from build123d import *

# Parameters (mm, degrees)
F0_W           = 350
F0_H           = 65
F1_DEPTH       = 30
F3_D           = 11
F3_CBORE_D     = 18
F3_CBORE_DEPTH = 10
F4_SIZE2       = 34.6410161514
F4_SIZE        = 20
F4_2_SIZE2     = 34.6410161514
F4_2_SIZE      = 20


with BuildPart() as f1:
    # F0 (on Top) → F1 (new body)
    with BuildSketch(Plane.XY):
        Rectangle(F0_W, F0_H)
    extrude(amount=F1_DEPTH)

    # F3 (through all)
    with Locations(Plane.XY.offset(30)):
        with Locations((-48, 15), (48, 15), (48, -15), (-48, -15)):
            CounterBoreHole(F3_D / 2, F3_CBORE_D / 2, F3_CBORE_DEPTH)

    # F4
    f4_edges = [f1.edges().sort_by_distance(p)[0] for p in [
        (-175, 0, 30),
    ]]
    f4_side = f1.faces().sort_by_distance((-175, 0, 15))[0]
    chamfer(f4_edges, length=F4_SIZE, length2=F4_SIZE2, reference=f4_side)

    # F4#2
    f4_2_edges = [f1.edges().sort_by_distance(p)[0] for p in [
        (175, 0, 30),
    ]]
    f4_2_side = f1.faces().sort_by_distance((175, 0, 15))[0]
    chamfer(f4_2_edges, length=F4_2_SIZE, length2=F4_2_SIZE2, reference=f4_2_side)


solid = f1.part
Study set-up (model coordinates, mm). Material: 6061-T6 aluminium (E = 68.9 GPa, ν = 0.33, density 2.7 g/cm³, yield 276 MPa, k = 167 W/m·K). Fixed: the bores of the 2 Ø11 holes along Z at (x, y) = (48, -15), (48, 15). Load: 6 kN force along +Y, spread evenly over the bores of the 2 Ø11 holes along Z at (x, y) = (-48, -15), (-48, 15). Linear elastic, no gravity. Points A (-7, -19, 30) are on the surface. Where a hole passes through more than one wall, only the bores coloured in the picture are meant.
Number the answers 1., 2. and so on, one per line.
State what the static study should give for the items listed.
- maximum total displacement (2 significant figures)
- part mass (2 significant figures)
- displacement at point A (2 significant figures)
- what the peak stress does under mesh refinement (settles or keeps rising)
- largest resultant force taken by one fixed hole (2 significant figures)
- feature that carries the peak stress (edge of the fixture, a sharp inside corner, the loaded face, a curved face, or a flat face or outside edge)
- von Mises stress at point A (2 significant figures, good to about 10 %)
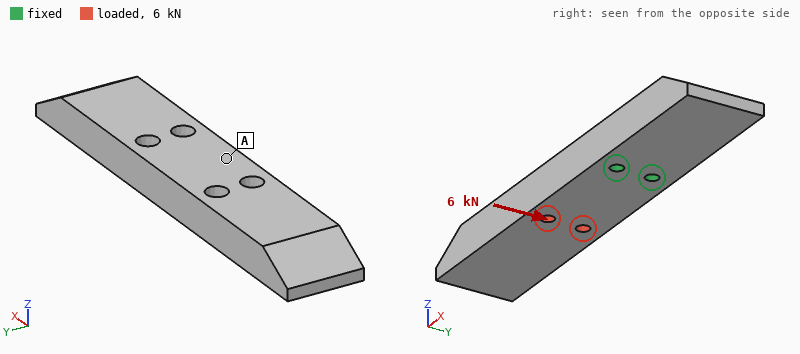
1. 0.17 mm
2. 1.7 kg
3. 0.031 mm
4. keeps rising
5. 16 kN
6. edge of the fixture
7. 6.5 MPa
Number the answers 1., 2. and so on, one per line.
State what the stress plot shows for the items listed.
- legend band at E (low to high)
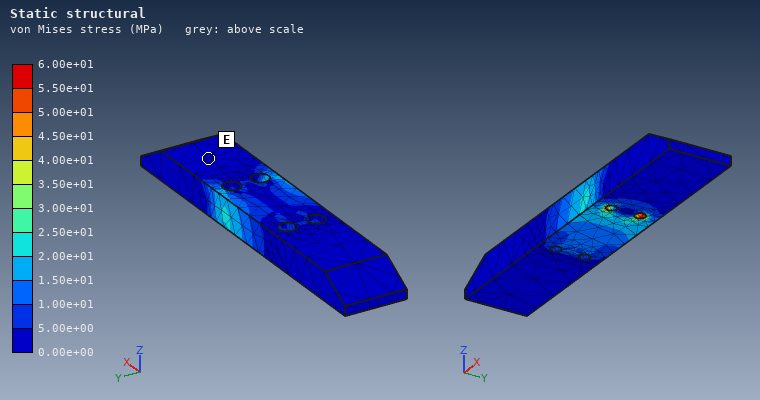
1. 0.00e+00 to 5.00e+00 MPa
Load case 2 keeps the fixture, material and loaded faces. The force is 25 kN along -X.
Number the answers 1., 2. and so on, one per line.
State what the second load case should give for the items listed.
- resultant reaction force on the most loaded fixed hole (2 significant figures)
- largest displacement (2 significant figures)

1. 13 kN
2. 0.19 mm
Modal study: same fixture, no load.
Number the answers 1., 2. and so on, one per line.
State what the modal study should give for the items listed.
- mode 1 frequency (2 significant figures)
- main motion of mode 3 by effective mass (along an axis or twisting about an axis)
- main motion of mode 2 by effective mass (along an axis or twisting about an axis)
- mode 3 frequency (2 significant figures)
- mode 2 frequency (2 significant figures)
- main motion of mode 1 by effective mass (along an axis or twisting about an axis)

1. 470 Hz
2. along Z
3. along Y
4. 1500 Hz
5. 980 Hz
6. along Z
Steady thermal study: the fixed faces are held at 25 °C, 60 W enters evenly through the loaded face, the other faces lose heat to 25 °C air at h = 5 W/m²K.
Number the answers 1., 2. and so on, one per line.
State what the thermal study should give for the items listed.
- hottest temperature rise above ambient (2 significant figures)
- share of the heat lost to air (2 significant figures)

1. 19 K
2. 5.2 %
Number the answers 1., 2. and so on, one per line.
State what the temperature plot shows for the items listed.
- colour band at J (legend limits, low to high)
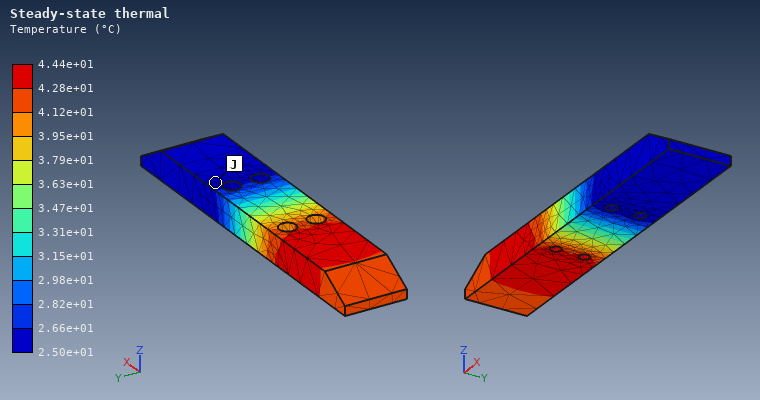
1. 2.50e+01 to 2.66e+01 °C
